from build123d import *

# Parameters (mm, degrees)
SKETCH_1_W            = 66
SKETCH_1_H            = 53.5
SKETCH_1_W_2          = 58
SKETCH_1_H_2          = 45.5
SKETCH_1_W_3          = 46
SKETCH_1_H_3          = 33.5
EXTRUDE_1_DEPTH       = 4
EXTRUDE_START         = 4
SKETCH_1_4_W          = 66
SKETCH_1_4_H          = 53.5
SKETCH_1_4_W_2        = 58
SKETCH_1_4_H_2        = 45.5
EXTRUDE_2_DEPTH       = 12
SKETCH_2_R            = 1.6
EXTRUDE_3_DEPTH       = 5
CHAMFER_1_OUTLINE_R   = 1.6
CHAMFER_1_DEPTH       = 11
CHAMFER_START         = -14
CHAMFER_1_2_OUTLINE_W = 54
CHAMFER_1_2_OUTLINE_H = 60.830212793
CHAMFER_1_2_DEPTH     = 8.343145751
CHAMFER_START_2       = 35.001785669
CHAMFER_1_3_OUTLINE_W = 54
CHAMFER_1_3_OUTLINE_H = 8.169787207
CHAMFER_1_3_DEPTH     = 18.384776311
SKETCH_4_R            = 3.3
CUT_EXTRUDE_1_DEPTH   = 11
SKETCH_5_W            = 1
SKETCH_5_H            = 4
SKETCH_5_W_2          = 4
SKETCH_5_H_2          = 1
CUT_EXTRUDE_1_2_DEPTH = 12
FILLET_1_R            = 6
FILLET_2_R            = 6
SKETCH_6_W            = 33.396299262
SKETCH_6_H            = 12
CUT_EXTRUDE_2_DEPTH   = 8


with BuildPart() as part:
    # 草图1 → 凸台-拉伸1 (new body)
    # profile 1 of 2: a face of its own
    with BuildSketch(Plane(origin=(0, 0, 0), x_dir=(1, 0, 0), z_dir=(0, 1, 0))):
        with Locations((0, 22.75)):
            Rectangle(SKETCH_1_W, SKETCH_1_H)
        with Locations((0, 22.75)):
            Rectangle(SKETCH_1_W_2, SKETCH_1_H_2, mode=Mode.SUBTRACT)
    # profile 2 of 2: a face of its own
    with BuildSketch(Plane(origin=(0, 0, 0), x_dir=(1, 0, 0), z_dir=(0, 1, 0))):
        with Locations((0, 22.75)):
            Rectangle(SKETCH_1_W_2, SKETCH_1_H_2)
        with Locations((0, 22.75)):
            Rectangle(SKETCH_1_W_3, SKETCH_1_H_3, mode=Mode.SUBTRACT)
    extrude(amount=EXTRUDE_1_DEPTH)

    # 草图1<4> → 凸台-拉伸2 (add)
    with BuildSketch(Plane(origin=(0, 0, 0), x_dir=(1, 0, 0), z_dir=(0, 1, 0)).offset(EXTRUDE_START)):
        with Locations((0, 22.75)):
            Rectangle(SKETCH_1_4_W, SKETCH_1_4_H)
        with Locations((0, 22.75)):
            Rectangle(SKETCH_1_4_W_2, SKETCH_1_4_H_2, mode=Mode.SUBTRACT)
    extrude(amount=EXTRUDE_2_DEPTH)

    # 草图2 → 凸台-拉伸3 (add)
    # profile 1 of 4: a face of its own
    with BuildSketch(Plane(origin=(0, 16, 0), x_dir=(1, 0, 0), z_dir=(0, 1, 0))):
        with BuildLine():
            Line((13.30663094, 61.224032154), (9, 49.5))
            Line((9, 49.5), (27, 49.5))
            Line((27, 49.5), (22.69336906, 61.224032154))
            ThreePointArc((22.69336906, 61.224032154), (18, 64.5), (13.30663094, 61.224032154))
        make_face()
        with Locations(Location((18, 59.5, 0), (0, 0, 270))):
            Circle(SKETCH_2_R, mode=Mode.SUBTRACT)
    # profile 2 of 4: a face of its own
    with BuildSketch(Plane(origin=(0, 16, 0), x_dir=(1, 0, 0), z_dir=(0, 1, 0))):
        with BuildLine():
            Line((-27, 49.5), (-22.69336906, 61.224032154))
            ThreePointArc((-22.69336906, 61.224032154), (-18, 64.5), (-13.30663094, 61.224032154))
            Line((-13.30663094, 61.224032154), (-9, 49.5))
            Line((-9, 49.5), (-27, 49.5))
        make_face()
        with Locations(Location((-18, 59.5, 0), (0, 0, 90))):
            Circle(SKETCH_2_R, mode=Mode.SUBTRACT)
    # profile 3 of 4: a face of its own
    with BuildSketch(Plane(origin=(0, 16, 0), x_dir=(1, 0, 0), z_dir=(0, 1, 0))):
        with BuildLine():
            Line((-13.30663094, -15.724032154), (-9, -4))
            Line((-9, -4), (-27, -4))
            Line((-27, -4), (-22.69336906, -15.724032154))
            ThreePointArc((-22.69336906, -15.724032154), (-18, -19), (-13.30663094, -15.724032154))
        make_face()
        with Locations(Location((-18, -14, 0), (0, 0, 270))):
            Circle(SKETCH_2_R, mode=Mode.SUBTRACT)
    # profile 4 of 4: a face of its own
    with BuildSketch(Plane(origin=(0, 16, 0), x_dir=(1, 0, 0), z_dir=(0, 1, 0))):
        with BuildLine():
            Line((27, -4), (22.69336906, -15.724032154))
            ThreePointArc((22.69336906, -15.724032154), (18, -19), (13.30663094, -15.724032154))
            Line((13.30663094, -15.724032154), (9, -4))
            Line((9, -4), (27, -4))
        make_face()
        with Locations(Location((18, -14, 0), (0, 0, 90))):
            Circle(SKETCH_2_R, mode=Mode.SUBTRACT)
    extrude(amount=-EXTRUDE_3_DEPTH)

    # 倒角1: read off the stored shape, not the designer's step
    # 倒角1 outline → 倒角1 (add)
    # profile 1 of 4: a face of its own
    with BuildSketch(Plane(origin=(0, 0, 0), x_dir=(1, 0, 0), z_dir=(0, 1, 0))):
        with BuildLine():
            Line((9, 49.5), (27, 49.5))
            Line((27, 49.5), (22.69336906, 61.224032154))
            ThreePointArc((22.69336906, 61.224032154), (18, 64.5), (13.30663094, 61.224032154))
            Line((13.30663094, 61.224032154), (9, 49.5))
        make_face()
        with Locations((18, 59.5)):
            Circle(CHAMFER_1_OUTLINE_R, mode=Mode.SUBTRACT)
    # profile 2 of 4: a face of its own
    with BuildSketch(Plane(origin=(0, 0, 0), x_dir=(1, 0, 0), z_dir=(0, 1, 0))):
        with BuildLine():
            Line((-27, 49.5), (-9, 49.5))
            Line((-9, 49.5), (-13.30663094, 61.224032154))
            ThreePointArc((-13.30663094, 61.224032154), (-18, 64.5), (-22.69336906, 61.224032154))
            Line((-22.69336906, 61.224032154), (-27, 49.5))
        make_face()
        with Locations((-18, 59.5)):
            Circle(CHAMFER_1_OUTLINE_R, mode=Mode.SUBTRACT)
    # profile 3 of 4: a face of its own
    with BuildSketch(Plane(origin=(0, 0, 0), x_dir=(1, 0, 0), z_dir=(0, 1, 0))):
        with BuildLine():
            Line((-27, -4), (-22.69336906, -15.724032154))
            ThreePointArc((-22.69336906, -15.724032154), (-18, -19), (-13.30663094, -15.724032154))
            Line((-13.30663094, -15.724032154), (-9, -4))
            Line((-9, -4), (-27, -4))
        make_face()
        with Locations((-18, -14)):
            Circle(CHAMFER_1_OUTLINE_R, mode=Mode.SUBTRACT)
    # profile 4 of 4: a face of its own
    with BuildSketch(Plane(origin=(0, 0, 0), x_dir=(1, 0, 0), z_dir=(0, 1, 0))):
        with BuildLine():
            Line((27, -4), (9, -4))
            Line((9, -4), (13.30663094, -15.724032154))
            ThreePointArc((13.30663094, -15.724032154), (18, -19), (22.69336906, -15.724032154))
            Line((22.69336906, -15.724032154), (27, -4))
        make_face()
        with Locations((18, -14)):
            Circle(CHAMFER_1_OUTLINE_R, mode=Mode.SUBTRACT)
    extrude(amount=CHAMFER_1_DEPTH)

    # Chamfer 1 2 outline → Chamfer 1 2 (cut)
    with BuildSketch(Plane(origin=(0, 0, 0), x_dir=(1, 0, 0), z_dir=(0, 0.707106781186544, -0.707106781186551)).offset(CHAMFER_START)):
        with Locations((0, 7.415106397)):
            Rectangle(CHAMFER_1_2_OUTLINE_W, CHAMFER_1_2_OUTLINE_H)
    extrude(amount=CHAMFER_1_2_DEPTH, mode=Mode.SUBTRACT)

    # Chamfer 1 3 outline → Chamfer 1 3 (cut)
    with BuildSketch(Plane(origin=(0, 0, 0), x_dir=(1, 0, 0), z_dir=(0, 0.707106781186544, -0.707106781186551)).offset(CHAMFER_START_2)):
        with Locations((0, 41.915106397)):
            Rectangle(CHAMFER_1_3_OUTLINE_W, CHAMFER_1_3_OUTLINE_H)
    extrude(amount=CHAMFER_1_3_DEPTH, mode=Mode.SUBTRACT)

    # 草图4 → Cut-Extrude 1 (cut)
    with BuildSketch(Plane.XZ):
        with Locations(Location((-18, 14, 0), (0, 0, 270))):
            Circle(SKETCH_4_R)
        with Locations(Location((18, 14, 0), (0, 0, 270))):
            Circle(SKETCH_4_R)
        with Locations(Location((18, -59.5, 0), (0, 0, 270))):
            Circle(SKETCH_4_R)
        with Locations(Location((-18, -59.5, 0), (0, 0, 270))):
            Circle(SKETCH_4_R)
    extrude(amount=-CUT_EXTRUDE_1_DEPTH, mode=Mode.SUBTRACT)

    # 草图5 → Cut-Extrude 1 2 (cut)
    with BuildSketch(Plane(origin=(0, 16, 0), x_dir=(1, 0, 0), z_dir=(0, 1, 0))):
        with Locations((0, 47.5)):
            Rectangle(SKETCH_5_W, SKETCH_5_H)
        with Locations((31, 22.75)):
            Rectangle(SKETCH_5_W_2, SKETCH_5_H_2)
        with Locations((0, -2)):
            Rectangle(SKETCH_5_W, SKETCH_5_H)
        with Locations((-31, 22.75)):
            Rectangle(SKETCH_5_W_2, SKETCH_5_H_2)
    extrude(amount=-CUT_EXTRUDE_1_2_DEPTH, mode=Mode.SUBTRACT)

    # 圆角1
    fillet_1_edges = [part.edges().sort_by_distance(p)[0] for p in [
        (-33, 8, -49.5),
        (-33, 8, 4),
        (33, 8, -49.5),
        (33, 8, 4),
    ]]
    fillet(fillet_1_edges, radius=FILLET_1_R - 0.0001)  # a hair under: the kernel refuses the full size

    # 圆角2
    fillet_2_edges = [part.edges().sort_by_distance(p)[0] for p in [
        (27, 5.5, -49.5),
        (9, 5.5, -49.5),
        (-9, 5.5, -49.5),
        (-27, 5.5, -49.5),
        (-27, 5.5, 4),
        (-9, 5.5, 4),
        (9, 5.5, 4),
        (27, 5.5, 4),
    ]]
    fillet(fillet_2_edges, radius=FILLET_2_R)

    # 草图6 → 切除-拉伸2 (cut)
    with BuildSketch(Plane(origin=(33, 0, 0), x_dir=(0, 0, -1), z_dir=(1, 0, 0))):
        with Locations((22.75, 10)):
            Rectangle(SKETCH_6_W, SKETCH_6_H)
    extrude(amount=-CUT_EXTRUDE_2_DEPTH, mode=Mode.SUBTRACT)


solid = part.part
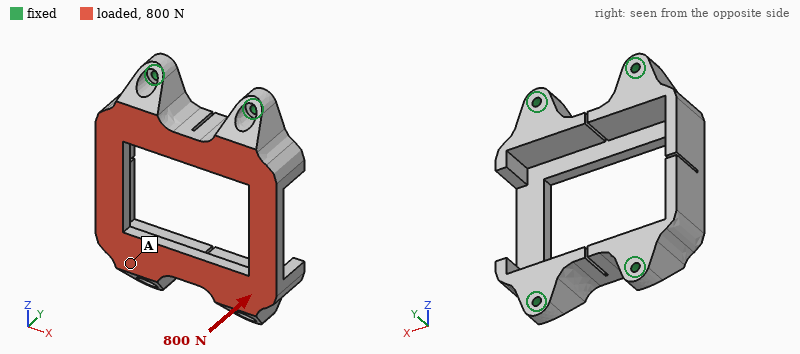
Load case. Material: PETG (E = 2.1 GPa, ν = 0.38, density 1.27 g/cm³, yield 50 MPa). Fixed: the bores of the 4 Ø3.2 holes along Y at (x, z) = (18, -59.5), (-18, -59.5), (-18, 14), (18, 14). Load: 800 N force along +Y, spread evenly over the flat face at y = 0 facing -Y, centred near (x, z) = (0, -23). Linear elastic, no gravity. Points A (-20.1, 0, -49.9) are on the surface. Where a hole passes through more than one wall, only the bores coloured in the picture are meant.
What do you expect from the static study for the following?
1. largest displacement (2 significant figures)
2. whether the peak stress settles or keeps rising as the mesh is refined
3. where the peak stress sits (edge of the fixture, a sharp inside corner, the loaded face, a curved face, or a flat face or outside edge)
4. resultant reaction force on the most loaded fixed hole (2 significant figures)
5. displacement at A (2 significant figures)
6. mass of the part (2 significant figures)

0.58 mm
keeps rising
edge of the fixture
280 N
0.16 mm
32 g
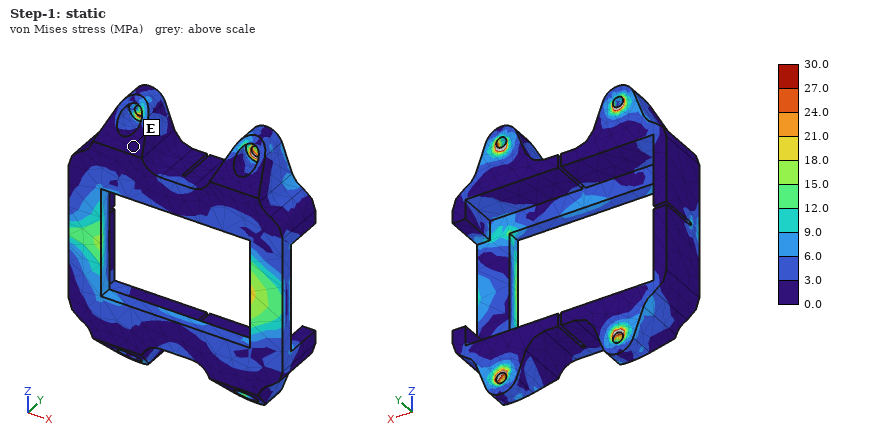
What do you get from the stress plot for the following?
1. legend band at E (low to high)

0.0 to 3.0 MPa
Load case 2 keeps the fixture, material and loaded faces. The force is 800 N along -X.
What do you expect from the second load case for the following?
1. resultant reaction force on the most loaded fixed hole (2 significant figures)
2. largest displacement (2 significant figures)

250 N
0.39 mm
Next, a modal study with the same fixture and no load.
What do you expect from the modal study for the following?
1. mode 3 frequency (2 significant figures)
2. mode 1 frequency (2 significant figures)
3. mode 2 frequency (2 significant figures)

1900 Hz
1600 Hz
1700 Hz
